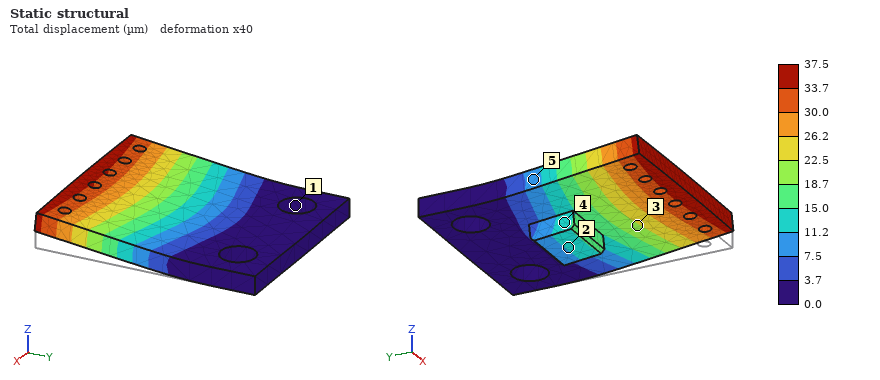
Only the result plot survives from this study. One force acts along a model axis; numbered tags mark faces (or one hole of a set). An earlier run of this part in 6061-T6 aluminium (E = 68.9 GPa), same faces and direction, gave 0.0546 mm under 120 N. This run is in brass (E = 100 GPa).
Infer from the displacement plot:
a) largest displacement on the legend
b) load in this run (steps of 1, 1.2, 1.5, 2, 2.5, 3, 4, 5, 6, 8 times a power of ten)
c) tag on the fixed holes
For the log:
37.5 µm
120 N
1
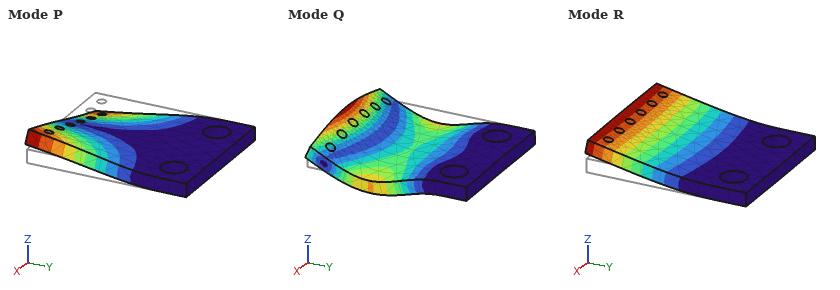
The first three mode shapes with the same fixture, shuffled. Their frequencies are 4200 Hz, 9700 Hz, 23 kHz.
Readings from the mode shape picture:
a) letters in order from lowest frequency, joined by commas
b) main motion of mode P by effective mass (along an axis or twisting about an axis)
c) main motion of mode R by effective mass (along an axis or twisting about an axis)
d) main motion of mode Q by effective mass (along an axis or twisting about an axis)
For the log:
R, P, Q
twisting about Y
along Z
along Z
